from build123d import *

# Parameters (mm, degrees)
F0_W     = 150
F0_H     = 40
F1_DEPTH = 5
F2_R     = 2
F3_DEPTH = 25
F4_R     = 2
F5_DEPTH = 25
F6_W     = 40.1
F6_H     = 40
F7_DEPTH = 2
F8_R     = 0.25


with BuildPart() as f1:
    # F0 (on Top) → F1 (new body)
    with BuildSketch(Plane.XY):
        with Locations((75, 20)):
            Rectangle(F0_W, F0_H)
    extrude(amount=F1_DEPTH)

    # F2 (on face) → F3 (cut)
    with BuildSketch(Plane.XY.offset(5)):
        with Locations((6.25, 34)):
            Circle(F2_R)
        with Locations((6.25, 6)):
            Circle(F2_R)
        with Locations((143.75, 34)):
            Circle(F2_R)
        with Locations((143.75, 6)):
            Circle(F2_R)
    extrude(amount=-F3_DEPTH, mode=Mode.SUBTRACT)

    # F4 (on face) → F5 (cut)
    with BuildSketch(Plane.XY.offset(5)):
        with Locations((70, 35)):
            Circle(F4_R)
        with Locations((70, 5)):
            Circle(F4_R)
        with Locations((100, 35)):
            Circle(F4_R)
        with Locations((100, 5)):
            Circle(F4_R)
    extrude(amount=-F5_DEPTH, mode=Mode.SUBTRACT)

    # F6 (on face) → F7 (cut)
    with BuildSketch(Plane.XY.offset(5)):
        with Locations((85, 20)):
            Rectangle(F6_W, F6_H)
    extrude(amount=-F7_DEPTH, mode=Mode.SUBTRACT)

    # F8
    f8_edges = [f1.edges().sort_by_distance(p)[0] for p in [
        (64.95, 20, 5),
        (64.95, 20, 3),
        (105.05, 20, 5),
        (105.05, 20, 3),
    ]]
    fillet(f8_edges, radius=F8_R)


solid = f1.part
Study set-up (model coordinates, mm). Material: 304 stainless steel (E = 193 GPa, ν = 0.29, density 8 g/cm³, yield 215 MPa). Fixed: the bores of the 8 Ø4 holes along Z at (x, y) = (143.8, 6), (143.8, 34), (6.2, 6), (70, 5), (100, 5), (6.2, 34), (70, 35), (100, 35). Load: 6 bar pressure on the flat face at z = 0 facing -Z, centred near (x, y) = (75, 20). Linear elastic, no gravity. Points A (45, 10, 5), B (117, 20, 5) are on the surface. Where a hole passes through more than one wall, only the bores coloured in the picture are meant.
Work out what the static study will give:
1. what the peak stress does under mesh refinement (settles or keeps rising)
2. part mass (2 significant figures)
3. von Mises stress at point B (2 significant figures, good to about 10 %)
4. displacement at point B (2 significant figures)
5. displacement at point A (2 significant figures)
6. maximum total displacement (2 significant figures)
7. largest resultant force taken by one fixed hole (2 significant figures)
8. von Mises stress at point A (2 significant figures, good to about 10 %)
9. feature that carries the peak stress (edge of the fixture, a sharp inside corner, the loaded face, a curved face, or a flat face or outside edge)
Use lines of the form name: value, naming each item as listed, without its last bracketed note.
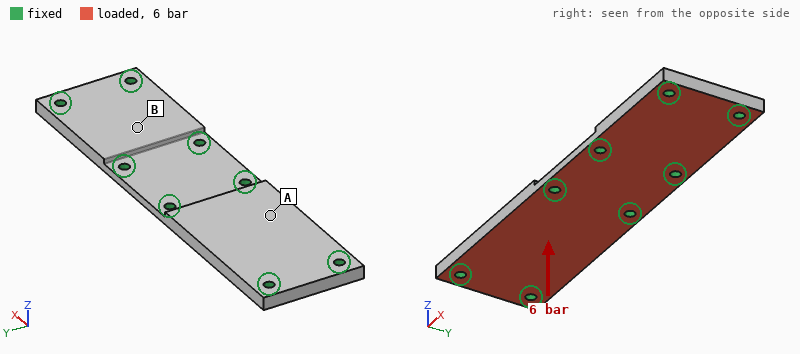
what the peak stress does under mesh refinement: keeps rising
part mass: 210 g
von Mises stress at point B: 11 MPa
displacement at point B: 5.1 µm
displacement at point A: 18 µm
maximum total displacement: 20 µm
largest resultant force taken by one fixed hole: 570 N
von Mises stress at point A: 29 MPa
feature that carries the peak stress: edge of the fixture
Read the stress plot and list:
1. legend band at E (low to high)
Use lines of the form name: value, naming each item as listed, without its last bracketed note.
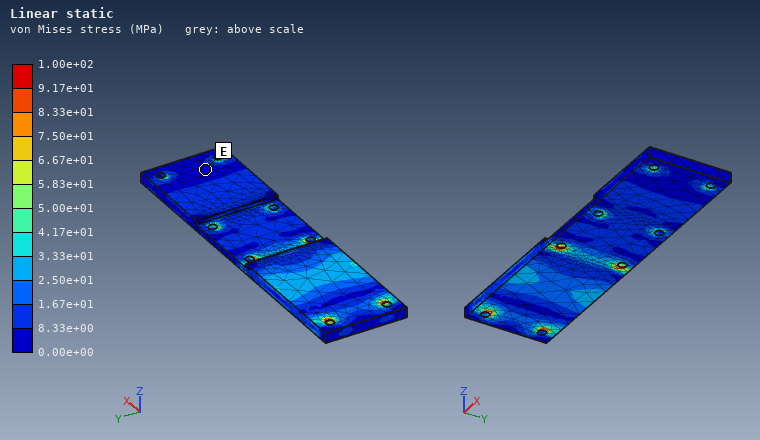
legend band at E: 0.00e+00 to 8.33e+00 MPa
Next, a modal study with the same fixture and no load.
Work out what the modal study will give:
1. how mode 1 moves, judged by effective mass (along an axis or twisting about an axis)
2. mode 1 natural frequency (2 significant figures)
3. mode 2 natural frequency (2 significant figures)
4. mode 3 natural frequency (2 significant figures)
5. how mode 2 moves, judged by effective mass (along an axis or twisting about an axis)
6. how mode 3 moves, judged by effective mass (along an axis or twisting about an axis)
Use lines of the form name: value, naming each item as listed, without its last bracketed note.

how mode 1 moves, judged by effective mass: along Z
mode 1 natural frequency: 5000 Hz
mode 2 natural frequency: 7900 Hz
mode 3 natural frequency: 9900 Hz
how mode 2 moves, judged by effective mass: twisting about X
how mode 3 moves, judged by effective mass: along Z
